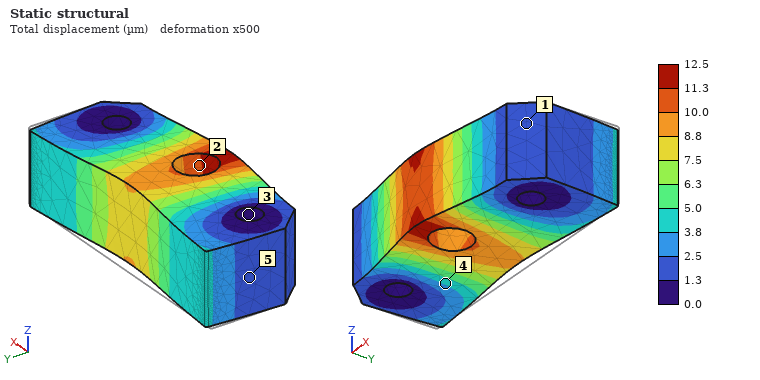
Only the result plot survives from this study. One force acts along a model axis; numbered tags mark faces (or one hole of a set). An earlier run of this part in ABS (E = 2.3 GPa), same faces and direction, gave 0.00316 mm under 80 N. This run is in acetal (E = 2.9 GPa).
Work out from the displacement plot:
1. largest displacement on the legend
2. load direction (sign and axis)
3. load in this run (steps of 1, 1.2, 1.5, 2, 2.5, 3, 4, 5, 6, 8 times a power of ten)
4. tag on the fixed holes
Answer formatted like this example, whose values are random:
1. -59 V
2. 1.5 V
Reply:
1. 12.5 µm
2. -Y
3. 400 N
4. 3
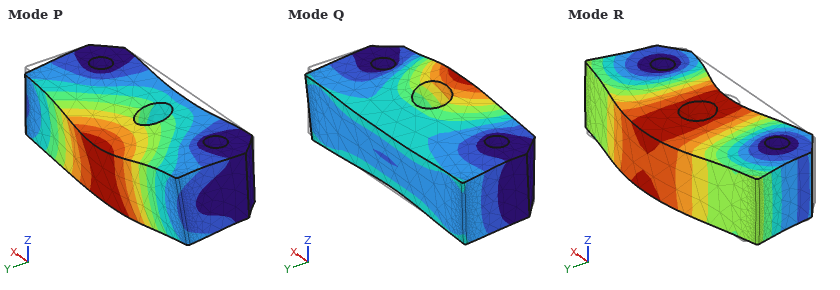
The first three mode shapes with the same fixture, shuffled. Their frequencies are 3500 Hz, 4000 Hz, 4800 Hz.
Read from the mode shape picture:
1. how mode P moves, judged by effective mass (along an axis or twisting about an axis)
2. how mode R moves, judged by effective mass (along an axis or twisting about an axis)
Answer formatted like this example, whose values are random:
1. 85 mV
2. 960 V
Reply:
1. along Z
2. along Y
